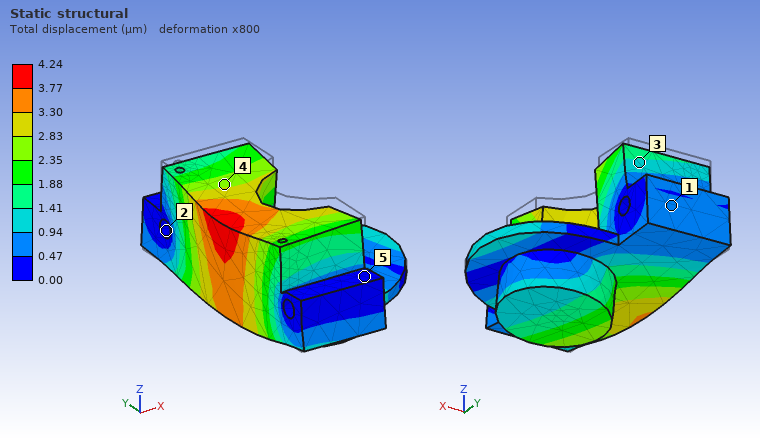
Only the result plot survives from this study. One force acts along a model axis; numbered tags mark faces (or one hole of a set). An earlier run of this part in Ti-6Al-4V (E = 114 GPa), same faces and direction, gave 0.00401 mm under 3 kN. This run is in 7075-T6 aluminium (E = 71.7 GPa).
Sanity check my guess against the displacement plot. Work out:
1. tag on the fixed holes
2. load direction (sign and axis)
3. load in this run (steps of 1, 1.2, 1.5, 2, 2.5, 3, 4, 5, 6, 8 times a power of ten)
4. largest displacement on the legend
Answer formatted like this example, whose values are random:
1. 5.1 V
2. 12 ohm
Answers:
1. 2
2. -Z
3. 2 kN
4. 4.24 µm
